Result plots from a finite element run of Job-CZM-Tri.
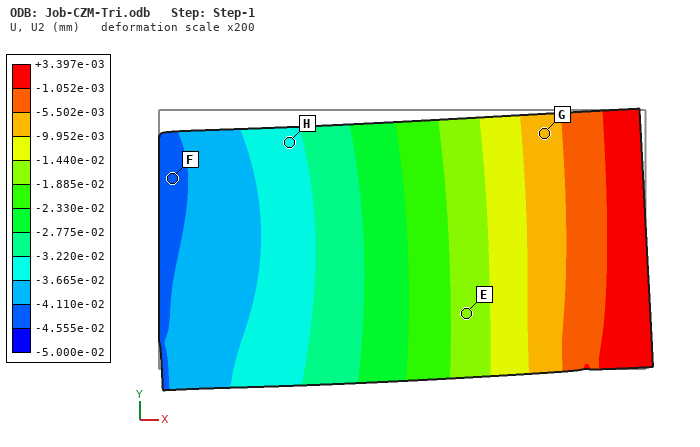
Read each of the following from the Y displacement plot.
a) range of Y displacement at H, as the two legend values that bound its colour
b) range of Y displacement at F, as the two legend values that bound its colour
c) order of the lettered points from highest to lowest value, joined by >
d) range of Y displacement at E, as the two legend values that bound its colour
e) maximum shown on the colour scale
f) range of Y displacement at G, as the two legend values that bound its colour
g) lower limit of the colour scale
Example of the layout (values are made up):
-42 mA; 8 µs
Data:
-3.665e-02 to -3.220e-02 mm; -4.555e-02 to -4.110e-02 mm; G > E > H > F; -1.885e-02 to -1.440e-02 mm; +3.397e-03 mm; -9.952e-03 to -5.502e-03 mm; -5.000e-02 mm
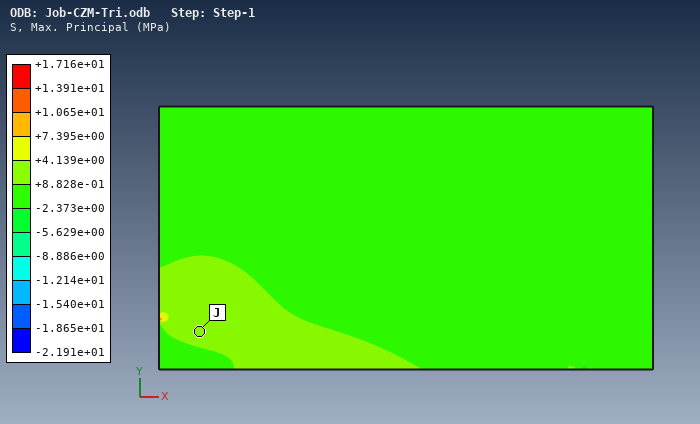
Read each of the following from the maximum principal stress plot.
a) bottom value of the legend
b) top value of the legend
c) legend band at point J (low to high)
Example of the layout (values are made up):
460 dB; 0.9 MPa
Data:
-2.191e+01 MPa; +1.716e+01 MPa; +8.828e-01 to +4.139e+00 MPa
